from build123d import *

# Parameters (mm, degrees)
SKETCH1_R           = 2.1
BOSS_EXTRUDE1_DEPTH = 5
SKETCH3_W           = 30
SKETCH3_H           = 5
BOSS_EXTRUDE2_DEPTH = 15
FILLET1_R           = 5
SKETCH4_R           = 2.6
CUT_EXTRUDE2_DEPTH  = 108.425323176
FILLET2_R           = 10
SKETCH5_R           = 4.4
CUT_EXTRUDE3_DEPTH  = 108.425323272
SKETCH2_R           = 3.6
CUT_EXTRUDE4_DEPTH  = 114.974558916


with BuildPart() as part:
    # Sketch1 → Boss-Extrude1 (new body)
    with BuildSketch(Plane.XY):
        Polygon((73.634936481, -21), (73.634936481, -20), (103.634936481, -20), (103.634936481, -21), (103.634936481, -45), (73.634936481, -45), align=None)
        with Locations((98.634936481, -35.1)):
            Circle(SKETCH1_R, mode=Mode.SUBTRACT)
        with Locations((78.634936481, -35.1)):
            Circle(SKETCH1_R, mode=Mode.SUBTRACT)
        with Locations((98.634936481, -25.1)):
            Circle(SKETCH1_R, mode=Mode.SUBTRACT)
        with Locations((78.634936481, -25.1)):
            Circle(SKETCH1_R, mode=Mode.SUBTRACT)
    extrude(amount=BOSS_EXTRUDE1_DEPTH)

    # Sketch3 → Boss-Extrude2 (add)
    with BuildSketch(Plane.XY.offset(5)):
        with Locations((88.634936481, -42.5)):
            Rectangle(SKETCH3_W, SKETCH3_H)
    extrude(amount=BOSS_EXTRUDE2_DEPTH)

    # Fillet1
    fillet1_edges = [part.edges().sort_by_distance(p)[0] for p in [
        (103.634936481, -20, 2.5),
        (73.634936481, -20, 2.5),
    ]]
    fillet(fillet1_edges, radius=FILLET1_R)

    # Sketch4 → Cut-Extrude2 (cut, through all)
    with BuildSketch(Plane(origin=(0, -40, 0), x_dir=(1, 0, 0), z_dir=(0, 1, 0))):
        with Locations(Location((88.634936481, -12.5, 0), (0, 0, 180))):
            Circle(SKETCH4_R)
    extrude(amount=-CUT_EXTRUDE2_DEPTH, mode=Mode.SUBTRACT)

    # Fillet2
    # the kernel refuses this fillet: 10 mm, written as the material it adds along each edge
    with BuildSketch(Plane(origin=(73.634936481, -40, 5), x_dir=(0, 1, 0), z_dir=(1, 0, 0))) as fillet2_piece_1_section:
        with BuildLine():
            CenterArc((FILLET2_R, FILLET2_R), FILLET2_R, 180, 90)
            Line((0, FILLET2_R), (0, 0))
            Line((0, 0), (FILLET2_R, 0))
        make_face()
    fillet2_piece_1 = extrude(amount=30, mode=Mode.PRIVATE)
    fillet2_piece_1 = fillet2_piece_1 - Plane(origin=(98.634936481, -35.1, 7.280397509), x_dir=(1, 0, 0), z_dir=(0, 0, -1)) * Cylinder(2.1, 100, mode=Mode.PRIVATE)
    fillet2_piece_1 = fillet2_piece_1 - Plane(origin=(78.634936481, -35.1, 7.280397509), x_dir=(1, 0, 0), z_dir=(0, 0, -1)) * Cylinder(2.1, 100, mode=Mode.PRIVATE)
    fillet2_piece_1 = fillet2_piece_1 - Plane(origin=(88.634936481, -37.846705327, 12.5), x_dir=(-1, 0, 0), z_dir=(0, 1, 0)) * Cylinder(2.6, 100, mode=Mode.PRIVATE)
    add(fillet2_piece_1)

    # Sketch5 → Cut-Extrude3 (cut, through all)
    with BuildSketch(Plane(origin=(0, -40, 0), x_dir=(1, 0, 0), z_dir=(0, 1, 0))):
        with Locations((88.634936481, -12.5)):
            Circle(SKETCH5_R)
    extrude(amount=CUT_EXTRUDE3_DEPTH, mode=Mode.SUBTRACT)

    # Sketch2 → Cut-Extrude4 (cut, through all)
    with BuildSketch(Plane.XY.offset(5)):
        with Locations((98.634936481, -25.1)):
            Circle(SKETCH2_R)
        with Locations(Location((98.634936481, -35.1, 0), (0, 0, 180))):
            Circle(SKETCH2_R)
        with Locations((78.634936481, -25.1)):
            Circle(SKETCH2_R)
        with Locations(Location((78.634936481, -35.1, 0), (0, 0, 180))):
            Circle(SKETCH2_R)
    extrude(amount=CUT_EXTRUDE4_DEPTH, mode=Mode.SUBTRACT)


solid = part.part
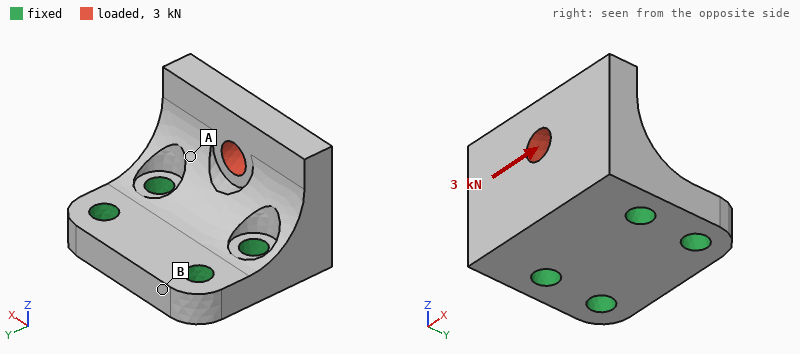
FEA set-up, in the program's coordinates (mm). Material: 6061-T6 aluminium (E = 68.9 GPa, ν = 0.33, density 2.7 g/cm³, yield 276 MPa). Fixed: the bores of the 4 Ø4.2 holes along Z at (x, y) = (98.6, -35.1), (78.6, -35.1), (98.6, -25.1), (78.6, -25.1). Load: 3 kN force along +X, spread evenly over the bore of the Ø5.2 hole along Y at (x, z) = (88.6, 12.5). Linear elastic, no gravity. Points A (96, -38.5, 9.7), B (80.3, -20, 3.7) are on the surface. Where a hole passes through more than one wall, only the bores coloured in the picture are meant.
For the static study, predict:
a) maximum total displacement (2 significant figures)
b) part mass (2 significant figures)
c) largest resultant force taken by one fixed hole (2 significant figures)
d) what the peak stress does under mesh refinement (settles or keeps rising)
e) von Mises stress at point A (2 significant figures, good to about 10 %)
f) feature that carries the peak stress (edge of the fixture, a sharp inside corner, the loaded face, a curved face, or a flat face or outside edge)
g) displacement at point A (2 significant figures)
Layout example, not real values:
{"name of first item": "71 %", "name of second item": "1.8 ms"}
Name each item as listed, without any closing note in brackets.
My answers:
{"maximum total displacement": "26 µm", "part mass": "16 g", "largest resultant force taken by one fixed hole": "2.1 kN", "what the peak stress does under mesh refinement": "keeps rising", "von Mises stress at point A": "41 MPa", "feature that carries the peak stress": "edge of the fixture", "displacement at point A": "11 µm"}
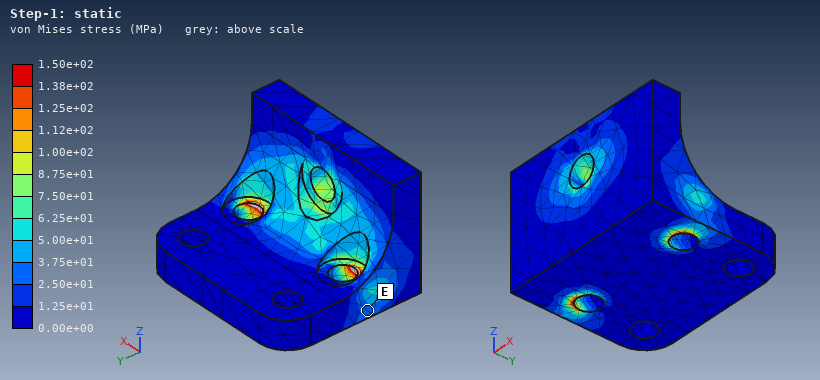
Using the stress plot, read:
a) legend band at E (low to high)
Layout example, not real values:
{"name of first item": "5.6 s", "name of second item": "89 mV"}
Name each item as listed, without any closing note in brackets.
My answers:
{"legend band at E": "2.50e+01 to 3.75e+01 MPa"}
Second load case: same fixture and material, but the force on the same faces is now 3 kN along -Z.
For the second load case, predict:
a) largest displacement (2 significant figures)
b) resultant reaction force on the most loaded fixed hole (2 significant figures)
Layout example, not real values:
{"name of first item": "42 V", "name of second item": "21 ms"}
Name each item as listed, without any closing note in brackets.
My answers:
{"largest displacement": "57 µm", "resultant reaction force on the most loaded fixed hole": "1.8 kN"}
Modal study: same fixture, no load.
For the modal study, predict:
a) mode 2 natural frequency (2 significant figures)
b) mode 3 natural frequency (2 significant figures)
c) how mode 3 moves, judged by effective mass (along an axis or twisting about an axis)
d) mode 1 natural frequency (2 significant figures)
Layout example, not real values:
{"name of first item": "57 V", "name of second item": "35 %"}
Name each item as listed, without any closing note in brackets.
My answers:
{"mode 2 natural frequency": "20 kHz", "mode 3 natural frequency": "28 kHz", "how mode 3 moves, judged by effective mass": "along X", "mode 1 natural frequency": "12 kHz"}
